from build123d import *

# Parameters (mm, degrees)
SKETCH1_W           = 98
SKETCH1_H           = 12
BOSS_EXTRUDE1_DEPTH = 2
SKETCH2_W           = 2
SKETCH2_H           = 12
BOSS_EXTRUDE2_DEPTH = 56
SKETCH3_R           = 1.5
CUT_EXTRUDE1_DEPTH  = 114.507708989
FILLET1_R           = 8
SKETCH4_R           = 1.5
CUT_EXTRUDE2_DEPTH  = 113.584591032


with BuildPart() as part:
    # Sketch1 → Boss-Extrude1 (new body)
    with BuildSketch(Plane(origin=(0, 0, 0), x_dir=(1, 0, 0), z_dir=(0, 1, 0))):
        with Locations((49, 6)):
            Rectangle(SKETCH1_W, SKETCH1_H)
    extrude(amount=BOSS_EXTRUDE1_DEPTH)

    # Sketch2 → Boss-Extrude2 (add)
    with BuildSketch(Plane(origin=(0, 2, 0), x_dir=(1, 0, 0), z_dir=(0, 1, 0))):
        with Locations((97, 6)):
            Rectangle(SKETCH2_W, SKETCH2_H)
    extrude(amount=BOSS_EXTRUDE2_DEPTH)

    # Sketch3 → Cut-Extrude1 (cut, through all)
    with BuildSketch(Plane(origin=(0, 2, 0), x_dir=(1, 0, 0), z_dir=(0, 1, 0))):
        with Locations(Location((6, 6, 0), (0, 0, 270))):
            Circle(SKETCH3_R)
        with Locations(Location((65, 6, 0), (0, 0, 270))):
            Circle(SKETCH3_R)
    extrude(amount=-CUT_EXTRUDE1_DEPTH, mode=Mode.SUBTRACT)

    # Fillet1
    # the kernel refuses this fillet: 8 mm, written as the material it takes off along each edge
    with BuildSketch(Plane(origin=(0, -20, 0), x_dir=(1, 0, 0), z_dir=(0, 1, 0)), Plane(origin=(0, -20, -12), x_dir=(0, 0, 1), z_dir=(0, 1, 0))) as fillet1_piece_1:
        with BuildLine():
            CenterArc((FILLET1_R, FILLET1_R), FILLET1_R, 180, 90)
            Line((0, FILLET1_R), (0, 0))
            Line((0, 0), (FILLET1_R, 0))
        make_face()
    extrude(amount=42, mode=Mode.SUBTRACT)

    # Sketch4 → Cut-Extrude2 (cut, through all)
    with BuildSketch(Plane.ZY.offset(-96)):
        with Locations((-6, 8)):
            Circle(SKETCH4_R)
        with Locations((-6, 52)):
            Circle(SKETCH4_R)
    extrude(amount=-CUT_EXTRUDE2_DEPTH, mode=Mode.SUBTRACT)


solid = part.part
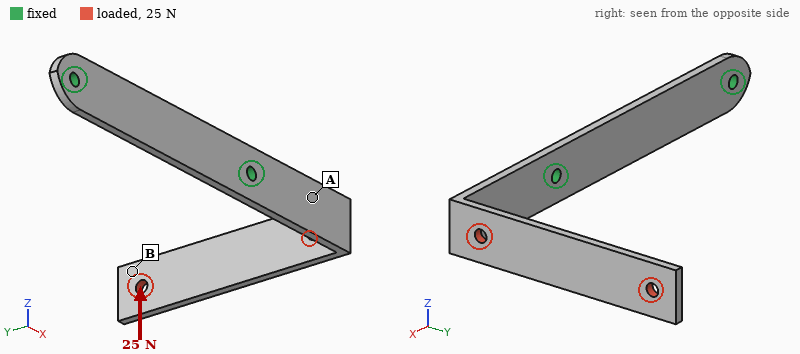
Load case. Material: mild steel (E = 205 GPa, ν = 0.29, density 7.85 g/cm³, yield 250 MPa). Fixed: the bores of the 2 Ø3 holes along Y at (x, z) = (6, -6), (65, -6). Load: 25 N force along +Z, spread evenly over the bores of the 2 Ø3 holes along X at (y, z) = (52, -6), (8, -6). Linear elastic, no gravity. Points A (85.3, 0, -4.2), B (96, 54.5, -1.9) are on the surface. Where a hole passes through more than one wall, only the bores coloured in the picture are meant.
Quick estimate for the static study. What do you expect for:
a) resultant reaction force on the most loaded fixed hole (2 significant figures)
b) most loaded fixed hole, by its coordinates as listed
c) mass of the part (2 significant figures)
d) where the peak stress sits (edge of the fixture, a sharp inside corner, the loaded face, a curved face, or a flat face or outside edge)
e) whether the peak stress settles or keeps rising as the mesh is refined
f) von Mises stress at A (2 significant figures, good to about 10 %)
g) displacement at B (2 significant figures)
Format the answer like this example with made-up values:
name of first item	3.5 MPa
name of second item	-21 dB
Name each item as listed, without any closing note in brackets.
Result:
resultant reaction force on the most loaded fixed hole	32 N
most loaded fixed hole, by its coordinates as listed	(65, -6)
mass of the part	28 g
where the peak stress sits	edge of the fixture
whether the peak stress settles or keeps rising as the mesh is refined	keeps rising
von Mises stress at A	84 MPa
displacement at B	0.52 mm
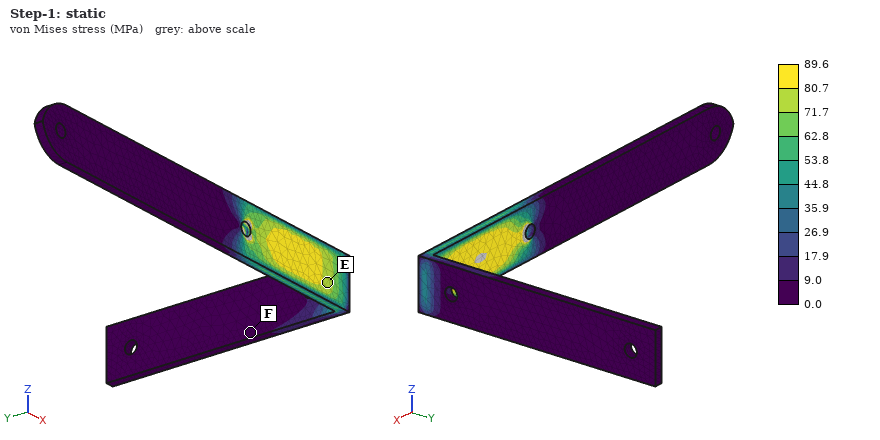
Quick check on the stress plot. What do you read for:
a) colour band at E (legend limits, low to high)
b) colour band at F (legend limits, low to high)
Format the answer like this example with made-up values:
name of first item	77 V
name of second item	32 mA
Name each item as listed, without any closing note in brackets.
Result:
colour band at E	71.7 to 80.7 MPa
colour band at F	0.0 to 9.0 MPa
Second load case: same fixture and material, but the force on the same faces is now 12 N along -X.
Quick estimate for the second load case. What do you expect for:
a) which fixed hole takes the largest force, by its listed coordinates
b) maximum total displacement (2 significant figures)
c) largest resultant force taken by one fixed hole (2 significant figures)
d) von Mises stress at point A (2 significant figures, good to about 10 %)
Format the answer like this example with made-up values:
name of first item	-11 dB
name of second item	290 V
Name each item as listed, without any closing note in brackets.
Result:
which fixed hole takes the largest force, by its listed coordinates	(65, -6)
maximum total displacement	0.58 mm
largest resultant force taken by one fixed hole	12 N
von Mises stress at point A	42 MPa
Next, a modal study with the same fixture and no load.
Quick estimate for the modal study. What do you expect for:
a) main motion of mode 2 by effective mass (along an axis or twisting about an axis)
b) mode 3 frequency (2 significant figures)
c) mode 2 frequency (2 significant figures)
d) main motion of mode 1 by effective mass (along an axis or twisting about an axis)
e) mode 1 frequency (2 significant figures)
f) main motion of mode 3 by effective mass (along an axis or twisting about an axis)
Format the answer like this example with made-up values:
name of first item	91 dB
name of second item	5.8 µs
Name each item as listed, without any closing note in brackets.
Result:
main motion of mode 2 by effective mass	along Z
mode 3 frequency	870 Hz
mode 2 frequency	410 Hz
main motion of mode 1 by effective mass	along X
mode 1 frequency	270 Hz
main motion of mode 3 by effective mass	along Y
